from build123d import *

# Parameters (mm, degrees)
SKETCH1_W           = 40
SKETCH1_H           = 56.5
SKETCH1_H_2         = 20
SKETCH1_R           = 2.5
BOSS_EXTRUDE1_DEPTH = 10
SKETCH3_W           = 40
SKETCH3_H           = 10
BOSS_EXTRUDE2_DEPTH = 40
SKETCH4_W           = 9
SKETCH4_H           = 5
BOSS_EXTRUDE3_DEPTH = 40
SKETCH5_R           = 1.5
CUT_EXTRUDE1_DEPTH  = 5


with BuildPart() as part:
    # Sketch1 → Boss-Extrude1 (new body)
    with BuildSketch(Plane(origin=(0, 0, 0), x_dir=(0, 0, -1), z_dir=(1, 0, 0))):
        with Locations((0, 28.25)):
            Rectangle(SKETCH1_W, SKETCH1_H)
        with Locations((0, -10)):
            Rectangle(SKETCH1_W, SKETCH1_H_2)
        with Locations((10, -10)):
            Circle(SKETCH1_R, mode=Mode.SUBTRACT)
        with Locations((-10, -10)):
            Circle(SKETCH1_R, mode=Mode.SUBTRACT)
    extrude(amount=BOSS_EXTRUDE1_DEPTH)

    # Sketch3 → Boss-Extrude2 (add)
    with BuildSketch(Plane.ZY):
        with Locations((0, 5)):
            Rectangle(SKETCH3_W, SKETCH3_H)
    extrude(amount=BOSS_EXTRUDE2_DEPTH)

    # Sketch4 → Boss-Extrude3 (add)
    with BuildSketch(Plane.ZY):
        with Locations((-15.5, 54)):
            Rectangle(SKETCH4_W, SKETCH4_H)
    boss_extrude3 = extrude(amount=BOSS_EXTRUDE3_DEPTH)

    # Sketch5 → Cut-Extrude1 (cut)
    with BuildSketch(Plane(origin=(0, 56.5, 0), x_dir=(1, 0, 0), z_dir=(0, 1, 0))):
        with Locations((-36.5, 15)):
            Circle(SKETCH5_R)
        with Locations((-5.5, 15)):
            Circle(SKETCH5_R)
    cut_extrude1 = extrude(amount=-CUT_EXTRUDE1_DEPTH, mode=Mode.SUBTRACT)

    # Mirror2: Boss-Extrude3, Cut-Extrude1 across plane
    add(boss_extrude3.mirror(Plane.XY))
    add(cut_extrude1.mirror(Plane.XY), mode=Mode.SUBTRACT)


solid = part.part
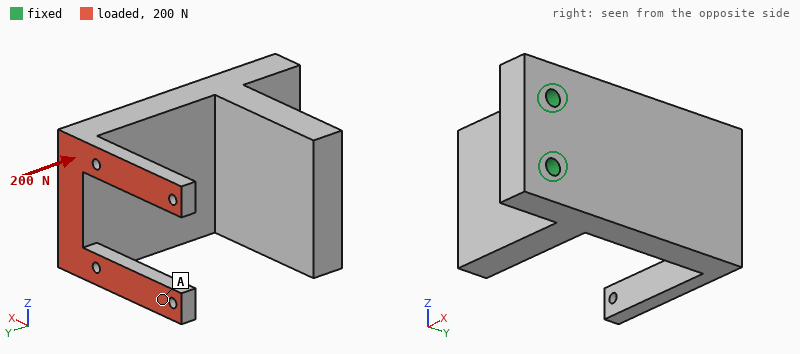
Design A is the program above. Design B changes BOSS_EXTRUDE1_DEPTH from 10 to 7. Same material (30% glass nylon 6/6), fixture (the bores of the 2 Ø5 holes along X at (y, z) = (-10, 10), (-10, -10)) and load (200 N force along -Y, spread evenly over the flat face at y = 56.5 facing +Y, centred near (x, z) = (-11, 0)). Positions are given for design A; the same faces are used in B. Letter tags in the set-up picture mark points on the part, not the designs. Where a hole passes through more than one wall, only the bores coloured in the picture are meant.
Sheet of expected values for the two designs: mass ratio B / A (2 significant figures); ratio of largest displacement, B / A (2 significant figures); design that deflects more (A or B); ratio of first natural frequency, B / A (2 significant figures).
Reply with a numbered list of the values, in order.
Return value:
1. 0.82
2. 1.6
3. B
4. 0.69
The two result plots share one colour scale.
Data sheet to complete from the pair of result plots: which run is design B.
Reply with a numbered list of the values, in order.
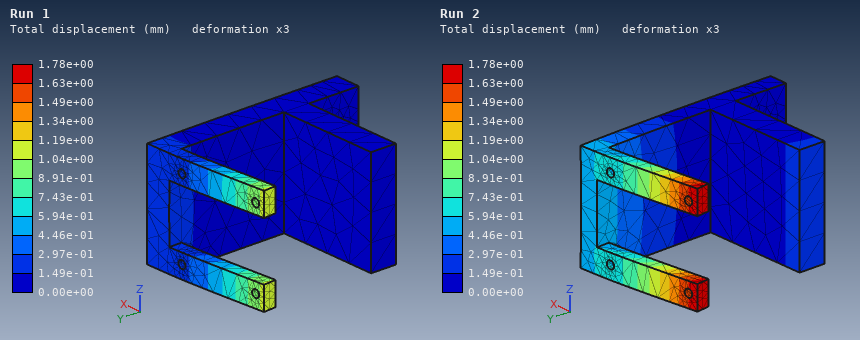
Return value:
1. Run 2
